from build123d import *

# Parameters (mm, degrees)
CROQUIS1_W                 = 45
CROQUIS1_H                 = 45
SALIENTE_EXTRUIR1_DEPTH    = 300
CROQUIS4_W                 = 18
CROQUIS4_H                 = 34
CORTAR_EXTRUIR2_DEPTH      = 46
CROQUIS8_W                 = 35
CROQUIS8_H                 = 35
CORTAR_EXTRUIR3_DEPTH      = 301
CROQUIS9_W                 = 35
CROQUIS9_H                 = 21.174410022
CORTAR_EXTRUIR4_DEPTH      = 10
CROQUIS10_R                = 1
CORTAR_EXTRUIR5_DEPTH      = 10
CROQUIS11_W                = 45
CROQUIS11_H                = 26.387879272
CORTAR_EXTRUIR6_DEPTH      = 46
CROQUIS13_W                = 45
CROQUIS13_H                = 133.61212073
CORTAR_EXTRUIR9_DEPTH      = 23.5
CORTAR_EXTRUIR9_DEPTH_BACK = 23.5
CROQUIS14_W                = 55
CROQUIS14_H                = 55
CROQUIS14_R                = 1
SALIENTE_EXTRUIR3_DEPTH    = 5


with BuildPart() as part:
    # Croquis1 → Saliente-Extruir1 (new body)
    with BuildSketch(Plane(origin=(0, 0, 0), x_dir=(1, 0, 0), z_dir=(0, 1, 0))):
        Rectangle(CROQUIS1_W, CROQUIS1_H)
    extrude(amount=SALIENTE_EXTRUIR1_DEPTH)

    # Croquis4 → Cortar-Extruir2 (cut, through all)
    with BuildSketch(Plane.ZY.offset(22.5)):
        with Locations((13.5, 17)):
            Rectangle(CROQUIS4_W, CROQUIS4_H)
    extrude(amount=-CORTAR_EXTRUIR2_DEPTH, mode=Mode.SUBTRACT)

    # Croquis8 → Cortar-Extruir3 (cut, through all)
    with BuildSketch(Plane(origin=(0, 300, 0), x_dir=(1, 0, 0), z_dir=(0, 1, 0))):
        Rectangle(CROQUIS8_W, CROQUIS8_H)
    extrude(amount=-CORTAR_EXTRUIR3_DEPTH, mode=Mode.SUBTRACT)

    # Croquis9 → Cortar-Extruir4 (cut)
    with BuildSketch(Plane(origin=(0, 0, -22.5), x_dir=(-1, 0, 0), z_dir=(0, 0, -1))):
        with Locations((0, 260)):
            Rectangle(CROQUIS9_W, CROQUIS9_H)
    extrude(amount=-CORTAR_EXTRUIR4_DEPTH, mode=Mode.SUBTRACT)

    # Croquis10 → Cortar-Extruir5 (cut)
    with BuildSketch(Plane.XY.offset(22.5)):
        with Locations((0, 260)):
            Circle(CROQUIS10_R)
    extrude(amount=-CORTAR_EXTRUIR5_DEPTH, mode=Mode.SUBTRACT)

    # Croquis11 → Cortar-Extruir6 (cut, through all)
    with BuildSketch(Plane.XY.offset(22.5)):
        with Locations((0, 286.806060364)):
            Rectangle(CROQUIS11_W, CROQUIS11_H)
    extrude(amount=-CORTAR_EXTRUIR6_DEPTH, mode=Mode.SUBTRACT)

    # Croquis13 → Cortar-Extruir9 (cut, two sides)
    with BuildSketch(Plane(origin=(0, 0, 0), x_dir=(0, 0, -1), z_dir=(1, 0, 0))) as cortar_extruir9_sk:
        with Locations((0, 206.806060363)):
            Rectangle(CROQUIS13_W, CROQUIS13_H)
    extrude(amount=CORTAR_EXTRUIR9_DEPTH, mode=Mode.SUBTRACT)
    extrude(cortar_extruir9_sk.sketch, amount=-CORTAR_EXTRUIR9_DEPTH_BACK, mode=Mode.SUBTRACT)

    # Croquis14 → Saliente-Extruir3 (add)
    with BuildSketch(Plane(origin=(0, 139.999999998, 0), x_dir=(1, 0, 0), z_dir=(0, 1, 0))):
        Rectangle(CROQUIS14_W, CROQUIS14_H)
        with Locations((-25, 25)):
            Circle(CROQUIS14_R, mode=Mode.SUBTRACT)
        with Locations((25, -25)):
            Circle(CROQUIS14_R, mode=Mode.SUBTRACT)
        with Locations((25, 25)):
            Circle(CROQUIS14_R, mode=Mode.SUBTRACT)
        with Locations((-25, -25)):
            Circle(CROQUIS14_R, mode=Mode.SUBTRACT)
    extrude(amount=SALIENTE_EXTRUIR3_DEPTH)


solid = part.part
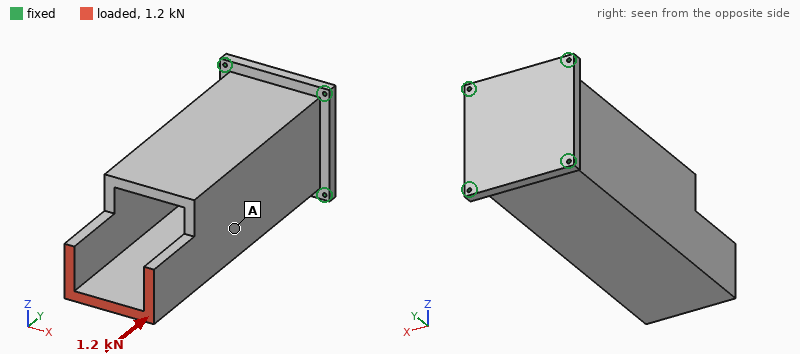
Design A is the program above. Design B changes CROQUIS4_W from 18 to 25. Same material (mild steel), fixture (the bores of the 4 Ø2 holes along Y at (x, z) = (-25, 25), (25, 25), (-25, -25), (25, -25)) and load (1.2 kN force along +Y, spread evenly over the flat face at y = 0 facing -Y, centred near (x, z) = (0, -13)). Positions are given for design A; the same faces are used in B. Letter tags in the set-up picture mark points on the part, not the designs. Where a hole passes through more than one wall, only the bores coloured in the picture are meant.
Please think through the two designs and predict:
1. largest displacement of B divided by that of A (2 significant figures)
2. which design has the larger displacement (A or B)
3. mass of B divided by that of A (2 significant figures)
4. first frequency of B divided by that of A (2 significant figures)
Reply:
1.1
B
0.99
1.0
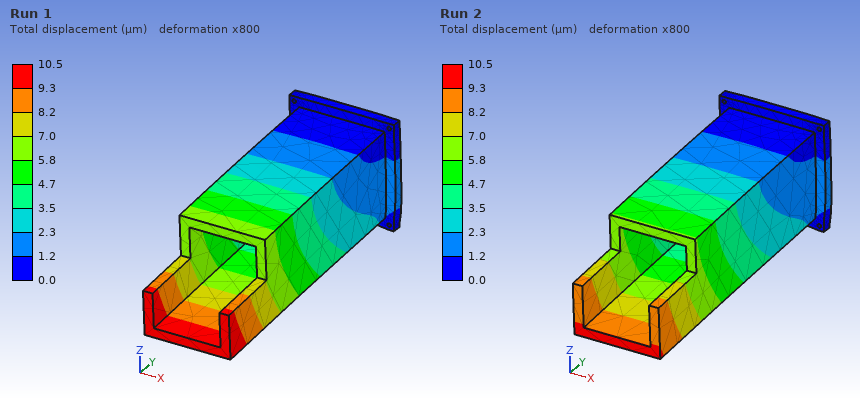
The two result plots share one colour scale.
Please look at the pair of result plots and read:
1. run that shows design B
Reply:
Run 1
